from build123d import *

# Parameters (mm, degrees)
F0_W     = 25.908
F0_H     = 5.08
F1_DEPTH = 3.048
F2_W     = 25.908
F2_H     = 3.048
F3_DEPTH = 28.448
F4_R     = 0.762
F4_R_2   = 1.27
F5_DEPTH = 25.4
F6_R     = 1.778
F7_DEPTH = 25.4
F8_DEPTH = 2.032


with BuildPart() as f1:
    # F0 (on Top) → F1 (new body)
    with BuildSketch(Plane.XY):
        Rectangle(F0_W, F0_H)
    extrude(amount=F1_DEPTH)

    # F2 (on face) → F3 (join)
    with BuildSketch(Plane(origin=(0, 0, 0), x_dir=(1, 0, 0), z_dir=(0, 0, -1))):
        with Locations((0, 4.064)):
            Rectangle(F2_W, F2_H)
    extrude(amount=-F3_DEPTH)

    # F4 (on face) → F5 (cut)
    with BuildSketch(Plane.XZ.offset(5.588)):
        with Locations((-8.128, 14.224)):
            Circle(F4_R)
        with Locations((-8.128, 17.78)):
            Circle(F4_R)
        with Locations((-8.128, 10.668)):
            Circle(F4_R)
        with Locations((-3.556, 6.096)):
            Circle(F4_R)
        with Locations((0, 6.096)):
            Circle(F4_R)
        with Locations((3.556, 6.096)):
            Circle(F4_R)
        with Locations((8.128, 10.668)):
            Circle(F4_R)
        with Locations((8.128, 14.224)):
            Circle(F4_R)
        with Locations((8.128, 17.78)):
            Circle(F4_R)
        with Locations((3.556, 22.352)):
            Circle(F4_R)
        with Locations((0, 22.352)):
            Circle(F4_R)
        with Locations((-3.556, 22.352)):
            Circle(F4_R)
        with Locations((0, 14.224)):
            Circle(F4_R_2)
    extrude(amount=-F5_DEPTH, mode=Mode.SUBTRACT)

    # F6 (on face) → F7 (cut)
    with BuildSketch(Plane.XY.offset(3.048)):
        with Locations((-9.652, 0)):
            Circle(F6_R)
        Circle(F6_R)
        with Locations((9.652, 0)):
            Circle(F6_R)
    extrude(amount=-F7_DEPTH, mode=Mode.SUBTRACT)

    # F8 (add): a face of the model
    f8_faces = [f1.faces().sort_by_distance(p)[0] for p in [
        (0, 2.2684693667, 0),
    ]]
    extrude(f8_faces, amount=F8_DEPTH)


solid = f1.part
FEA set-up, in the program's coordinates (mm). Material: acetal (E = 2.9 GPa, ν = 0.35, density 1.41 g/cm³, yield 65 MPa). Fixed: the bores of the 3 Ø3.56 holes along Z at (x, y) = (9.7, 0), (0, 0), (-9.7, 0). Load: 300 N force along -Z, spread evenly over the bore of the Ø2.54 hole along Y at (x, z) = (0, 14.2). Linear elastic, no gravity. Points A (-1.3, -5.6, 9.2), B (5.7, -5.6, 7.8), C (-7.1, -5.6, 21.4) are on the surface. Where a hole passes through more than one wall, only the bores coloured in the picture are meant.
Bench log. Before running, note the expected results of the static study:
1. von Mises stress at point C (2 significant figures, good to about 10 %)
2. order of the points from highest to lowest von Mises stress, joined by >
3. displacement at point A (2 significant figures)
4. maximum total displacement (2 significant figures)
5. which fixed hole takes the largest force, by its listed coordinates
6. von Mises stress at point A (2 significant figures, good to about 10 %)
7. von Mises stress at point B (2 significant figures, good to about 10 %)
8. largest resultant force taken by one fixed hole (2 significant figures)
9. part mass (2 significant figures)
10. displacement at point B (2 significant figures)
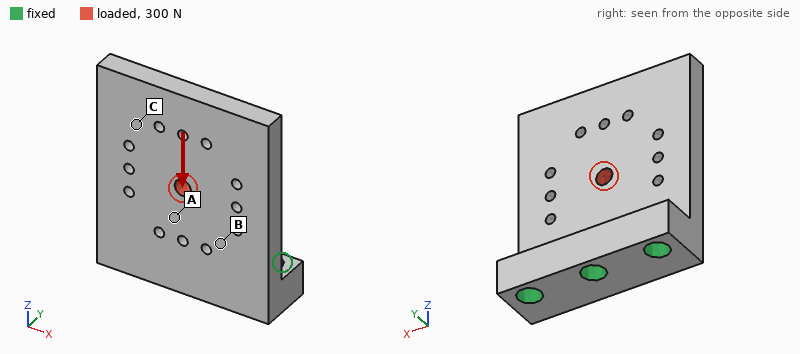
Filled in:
1.7 MPa
A > B > C
0.046 mm
0.11 mm
(0, 0)
7.5 MPa
4.9 MPa
110 N
4.0 g
0.036 mm
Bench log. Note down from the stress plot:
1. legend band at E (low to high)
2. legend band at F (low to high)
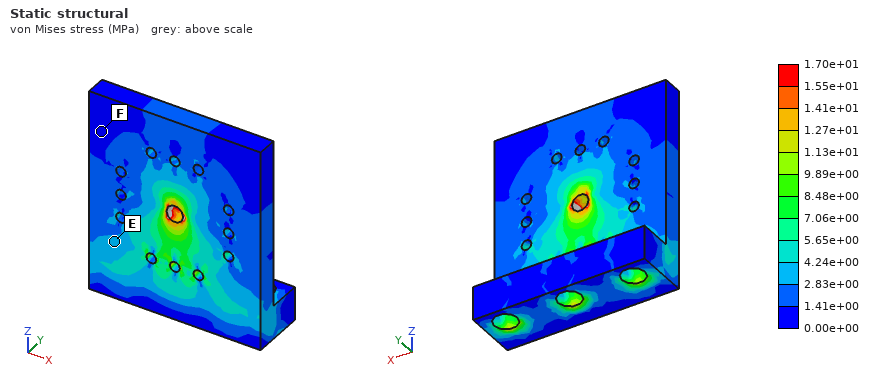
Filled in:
2.83e+00 to 4.24e+00 MPa
0.00e+00 to 1.41e+00 MPa
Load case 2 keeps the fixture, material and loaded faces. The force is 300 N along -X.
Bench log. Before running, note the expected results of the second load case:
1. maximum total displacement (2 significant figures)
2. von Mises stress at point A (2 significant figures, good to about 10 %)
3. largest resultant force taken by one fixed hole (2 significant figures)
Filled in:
0.18 mm
7.3 MPa
210 N
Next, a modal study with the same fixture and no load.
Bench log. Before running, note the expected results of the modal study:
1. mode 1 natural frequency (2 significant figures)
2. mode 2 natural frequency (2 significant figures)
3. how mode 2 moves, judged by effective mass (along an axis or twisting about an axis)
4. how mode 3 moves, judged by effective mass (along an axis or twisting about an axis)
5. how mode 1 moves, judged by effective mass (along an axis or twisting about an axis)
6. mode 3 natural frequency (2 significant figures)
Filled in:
940 Hz
2200 Hz
twisting about Z
along X
along Y
4400 Hz
